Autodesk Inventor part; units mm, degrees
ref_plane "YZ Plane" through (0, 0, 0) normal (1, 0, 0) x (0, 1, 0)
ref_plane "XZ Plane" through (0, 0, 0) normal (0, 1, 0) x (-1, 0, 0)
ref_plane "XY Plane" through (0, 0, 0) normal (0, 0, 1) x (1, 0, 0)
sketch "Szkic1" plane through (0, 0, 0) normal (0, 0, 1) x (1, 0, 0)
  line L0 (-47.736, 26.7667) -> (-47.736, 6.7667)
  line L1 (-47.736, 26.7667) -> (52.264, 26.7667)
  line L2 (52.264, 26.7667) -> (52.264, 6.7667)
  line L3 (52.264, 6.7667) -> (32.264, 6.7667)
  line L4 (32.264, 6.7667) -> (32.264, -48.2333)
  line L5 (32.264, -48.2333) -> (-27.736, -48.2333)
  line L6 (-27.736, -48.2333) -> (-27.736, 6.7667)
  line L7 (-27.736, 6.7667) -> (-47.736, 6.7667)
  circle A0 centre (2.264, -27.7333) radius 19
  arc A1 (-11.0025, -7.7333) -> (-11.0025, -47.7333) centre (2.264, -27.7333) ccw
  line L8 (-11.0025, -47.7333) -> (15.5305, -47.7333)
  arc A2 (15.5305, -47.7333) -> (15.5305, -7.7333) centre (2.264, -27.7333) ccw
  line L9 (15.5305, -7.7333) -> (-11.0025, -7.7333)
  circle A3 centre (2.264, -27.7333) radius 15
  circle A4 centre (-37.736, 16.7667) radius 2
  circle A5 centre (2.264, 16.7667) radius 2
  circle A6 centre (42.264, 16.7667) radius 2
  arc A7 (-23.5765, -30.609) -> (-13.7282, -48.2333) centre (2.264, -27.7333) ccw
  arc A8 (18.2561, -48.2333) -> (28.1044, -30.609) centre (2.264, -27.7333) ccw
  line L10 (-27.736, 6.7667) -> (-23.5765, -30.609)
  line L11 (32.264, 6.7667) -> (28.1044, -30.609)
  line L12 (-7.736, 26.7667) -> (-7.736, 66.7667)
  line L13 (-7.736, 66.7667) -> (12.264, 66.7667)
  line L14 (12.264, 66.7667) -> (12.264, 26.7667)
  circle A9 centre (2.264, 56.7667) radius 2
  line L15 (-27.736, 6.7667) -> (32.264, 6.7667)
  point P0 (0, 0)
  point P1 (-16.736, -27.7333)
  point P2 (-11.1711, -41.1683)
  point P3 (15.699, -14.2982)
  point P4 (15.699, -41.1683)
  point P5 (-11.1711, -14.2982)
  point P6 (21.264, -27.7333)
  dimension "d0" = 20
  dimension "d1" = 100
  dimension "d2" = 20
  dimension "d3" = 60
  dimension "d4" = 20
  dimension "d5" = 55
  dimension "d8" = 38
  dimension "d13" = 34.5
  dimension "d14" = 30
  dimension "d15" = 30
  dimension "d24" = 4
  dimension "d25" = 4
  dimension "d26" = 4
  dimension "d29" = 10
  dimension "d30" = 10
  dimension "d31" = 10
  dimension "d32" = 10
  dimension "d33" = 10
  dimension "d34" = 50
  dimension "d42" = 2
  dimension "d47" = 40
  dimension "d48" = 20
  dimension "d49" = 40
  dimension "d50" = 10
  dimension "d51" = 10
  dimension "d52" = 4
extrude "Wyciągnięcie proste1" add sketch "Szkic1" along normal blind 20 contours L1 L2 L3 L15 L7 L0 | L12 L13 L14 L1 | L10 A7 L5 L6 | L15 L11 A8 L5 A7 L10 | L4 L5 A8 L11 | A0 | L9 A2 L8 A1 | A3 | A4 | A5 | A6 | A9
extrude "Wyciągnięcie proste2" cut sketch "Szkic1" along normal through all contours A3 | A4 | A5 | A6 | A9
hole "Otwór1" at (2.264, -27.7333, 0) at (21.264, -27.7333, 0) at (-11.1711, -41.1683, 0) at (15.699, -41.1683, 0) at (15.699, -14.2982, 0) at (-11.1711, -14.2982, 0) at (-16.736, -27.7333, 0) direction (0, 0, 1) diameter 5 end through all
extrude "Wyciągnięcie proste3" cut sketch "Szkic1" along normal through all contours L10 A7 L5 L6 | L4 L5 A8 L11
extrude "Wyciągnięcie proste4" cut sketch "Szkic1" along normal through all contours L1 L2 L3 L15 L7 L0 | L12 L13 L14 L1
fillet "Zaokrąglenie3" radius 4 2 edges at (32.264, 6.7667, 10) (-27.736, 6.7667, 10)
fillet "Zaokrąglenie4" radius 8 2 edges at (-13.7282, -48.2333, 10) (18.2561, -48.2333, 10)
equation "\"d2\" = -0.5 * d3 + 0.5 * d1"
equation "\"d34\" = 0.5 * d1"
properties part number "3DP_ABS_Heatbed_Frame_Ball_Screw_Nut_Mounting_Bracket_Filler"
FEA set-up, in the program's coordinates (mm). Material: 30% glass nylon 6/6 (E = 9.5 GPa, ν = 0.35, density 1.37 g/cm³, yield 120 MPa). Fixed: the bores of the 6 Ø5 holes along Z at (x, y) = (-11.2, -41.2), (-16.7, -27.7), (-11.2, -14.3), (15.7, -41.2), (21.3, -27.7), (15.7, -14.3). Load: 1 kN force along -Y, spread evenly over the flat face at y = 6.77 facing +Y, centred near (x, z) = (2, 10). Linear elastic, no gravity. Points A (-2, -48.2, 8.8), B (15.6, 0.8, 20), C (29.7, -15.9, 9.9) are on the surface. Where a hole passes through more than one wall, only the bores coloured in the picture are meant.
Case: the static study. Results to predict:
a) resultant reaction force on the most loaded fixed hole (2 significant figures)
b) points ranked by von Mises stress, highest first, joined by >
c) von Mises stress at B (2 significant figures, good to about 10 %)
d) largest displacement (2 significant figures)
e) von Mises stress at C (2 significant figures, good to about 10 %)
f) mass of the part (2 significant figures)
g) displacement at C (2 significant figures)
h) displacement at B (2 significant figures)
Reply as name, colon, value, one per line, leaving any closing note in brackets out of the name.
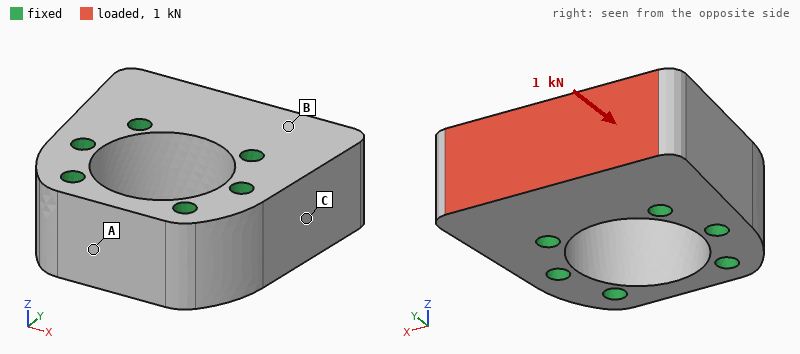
resultant reaction force on the most loaded fixed hole: 430 N
points ranked by von Mises stress, highest first, joined by >: B > C > A
von Mises stress at B: 1.1 MPa
largest displacement: 3.0 µm
von Mises stress at C: 0.61 MPa
mass of the part: 56 g
displacement at C: 0.99 µm
displacement at B: 2.1 µm
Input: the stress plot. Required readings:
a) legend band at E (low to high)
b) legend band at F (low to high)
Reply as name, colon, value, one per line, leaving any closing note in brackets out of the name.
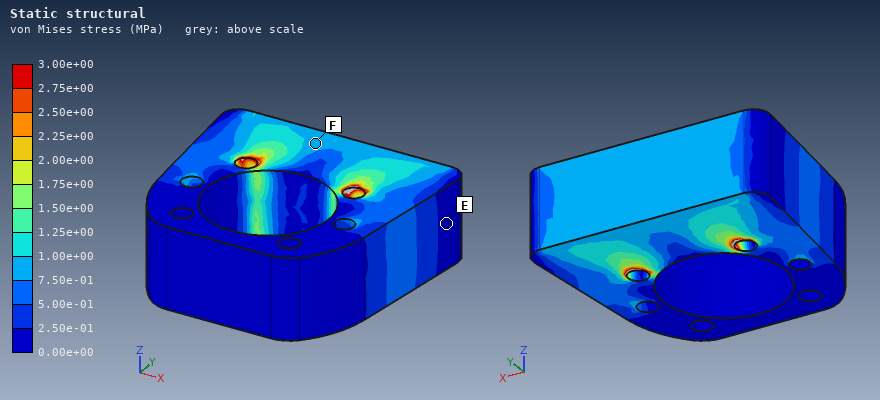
legend band at E: 0.00e+00 to 2.50e-01 MPa
legend band at F: 7.50e-01 to 1.00e+00 MPa
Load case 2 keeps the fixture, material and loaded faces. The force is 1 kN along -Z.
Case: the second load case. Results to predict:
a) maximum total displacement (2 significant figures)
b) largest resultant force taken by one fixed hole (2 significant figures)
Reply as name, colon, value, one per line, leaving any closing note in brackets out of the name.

maximum total displacement: 25 µm
largest resultant force taken by one fixed hole: 550 N
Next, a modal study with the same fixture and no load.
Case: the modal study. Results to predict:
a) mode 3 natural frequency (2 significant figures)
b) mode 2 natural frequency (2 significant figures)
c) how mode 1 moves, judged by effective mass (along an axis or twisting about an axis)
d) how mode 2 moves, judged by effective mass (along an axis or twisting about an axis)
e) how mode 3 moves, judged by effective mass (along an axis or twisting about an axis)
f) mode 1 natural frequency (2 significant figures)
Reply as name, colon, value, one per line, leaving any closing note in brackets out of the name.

mode 3 natural frequency: 13 kHz
mode 2 natural frequency: 12 kHz
how mode 1 moves, judged by effective mass: along Z
how mode 2 moves, judged by effective mass: twisting about Y
how mode 3 moves, judged by effective mass: along X
mode 1 natural frequency: 10 kHz
